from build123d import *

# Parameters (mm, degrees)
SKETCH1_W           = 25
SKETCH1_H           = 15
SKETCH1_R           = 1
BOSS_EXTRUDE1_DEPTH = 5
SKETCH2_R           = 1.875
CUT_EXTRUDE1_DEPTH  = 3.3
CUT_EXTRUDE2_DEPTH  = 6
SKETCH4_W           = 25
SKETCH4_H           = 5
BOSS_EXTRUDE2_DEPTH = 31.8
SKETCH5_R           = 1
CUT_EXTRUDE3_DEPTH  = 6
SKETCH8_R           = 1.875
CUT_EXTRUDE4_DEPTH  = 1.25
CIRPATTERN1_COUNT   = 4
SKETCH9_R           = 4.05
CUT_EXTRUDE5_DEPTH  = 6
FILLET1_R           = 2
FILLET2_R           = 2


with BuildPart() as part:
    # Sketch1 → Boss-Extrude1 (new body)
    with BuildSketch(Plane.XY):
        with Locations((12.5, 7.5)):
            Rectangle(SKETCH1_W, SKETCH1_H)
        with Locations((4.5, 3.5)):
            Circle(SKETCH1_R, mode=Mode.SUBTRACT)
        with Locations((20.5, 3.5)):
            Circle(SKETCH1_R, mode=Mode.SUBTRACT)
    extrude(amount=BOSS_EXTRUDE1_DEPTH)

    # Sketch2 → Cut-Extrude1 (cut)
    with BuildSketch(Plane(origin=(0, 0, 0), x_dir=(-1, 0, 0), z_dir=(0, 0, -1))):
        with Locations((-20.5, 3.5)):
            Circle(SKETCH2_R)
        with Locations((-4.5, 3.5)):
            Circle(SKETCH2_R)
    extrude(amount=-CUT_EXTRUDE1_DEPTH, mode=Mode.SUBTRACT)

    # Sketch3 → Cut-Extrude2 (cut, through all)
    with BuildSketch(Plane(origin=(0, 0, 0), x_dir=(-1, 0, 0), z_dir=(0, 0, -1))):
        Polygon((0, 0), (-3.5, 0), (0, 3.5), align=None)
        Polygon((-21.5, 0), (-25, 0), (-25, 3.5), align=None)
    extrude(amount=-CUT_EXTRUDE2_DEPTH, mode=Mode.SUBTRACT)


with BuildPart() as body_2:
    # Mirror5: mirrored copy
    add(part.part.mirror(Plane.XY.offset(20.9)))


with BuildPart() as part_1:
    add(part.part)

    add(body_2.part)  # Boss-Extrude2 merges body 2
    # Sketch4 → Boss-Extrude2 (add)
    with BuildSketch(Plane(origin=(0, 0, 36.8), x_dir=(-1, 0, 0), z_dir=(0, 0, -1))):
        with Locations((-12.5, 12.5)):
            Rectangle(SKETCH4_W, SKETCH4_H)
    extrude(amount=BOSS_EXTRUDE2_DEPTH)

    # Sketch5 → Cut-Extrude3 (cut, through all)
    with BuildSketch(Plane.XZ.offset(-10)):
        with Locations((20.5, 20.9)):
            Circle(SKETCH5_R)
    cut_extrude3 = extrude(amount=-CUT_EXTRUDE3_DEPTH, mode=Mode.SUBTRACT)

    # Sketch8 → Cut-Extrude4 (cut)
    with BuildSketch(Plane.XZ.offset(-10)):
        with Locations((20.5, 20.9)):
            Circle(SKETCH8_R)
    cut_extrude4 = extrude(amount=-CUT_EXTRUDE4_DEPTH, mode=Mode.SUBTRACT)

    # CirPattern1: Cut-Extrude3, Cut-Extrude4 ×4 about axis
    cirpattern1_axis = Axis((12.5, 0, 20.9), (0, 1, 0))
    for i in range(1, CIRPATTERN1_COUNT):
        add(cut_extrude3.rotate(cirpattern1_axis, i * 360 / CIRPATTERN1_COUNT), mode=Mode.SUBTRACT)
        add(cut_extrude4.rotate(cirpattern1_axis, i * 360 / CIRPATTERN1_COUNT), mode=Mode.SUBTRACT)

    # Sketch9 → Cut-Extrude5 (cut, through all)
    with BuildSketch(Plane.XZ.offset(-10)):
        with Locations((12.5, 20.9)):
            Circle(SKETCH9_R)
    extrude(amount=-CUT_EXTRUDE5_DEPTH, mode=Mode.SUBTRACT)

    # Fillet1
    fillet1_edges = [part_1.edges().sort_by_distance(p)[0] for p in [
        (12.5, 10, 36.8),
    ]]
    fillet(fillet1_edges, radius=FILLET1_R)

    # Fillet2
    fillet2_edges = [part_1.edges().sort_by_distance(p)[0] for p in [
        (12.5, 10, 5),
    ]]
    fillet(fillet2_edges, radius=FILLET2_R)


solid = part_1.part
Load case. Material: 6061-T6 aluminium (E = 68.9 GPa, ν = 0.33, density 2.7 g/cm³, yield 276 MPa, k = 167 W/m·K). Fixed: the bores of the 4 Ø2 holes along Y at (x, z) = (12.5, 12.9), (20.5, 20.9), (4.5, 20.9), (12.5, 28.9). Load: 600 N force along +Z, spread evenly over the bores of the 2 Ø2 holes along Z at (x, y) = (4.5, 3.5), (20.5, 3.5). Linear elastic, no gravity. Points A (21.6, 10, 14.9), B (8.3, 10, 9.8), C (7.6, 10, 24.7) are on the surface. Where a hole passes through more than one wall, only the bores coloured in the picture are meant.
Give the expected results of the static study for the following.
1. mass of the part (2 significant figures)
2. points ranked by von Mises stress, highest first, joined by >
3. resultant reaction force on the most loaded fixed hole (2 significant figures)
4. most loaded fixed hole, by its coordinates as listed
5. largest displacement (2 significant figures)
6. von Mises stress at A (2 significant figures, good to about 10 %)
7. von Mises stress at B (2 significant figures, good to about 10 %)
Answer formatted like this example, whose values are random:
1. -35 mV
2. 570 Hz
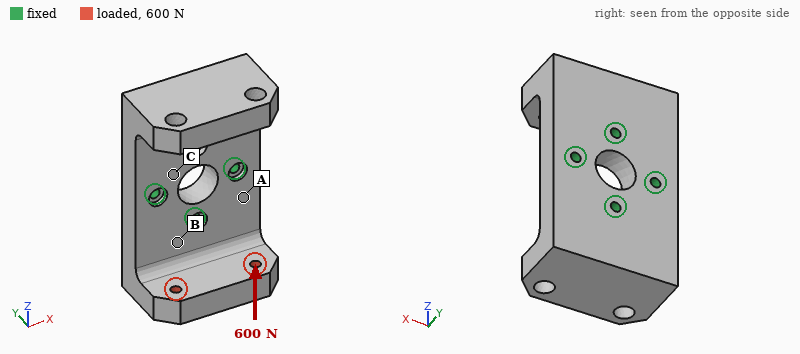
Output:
1. 19 g
2. B > A > C
3. 430 N
4. (12.5, 12.9)
5. 67 µm
6. 36 MPa
7. 53 MPa
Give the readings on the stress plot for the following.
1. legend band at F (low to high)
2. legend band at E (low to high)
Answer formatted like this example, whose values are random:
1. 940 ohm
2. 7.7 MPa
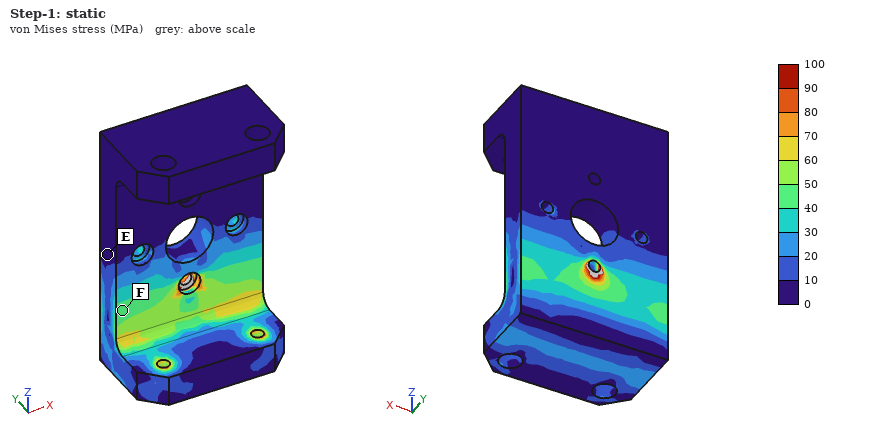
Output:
1. 40 to 50 MPa
2. 0 to 10 MPa
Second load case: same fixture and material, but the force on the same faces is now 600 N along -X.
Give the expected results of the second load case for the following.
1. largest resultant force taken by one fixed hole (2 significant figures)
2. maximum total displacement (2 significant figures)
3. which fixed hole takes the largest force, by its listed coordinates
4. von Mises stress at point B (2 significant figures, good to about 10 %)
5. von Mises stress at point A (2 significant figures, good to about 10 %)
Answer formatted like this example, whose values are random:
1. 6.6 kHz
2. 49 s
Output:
1. 530 N
2. 43 µm
3. (12.5, 12.9)
4. 42 MPa
5. 27 MPa
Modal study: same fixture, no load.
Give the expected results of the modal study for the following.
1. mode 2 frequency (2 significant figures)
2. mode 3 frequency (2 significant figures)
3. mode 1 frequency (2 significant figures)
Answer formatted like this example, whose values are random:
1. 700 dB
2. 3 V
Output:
1. 8200 Hz
2. 10 kHz
3. 8100 Hz
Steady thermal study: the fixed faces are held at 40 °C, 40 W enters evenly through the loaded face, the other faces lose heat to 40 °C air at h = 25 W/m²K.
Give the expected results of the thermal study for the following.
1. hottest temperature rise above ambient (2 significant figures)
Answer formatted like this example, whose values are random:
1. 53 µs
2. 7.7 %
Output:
1. 55 K
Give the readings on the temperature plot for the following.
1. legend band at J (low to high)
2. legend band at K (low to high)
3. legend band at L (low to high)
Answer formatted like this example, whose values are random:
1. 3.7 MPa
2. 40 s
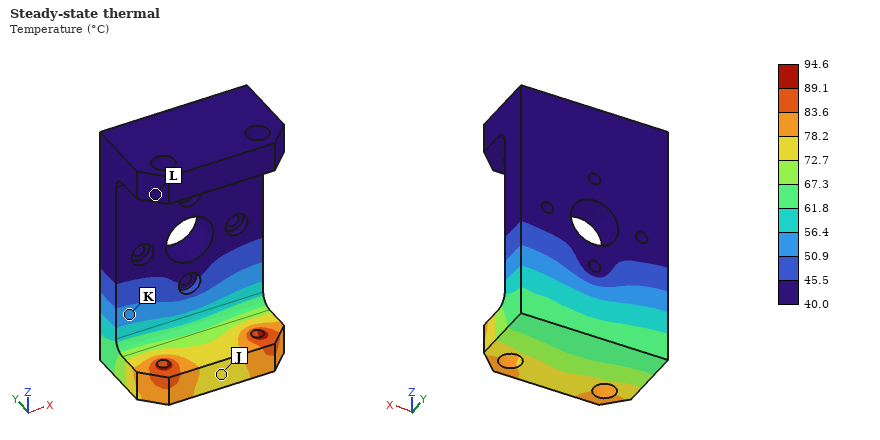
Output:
1. 72.7 to 78.2 °C
2. 50.9 to 56.4 °C
3. 40.0 to 45.5 °C
